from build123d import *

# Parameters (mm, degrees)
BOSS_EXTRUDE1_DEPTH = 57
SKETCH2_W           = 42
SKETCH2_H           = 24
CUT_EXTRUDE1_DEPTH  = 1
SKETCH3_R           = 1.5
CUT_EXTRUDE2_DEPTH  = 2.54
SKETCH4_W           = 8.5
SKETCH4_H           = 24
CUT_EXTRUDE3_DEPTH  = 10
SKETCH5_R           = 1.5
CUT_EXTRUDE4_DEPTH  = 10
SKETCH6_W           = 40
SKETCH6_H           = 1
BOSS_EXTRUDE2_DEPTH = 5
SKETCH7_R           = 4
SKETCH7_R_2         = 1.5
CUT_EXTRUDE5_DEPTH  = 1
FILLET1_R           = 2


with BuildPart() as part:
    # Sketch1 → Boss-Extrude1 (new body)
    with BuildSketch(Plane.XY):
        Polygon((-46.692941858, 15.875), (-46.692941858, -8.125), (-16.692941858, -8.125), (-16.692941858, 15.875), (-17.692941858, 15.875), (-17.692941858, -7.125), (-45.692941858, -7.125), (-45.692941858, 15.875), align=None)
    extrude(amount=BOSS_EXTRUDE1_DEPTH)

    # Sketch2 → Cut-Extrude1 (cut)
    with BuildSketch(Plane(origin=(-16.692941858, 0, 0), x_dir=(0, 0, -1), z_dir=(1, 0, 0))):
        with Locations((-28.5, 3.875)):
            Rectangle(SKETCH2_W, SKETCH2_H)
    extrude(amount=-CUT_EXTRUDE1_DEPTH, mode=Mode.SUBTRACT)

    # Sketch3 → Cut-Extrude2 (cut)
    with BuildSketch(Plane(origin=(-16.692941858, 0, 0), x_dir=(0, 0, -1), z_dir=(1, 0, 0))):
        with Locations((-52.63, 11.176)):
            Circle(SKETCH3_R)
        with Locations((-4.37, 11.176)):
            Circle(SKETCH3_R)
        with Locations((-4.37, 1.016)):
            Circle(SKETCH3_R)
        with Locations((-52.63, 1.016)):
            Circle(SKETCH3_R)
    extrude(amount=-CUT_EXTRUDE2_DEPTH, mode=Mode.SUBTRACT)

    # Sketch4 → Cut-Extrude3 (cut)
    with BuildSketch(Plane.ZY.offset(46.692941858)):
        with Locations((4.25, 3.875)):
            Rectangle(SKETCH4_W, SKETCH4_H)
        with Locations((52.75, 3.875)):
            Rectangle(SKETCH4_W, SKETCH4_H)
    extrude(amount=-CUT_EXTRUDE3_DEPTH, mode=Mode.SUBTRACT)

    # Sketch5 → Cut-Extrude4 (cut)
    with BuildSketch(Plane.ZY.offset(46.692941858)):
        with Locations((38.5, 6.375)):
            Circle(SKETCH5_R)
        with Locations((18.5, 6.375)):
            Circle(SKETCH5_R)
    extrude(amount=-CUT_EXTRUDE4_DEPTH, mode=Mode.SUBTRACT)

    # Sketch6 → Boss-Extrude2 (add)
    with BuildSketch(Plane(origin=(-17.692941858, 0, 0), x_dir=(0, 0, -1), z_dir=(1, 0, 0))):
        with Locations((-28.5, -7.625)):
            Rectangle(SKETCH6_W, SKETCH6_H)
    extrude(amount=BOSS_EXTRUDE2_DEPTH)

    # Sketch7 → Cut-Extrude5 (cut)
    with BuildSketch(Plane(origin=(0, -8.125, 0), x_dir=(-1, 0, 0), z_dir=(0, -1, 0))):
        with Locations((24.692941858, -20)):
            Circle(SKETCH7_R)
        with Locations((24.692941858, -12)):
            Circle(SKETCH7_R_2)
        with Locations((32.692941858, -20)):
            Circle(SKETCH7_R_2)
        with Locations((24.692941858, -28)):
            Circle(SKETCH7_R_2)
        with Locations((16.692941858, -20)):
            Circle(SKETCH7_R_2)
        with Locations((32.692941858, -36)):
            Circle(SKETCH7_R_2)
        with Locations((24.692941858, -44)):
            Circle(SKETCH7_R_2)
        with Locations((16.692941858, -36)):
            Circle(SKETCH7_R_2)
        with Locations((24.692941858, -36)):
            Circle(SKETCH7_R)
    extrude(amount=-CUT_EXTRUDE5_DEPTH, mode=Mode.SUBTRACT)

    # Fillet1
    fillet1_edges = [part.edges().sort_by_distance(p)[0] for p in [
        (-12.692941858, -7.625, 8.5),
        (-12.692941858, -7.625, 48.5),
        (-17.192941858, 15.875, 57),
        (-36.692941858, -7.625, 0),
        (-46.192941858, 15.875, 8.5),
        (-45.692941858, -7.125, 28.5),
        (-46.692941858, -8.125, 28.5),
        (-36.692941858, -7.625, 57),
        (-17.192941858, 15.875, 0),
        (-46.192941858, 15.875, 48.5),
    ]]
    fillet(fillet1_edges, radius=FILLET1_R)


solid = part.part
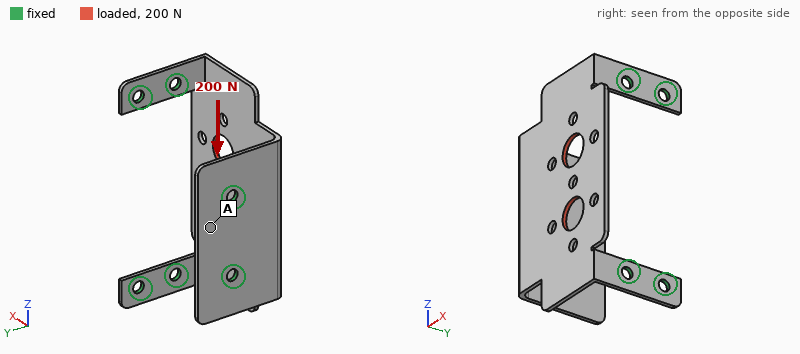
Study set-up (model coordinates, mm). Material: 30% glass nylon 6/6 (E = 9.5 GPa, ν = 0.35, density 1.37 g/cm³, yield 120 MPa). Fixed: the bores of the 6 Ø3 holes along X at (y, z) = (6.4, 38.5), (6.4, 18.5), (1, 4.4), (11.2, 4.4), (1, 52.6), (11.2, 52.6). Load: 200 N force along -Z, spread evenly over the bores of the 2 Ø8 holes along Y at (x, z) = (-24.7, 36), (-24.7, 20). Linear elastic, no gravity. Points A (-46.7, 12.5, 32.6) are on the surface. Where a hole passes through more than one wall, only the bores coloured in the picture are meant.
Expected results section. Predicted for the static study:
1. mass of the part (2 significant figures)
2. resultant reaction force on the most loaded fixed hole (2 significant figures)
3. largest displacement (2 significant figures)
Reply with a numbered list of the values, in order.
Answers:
1. 3.8 g
2. 89 N
3. 0.15 mm
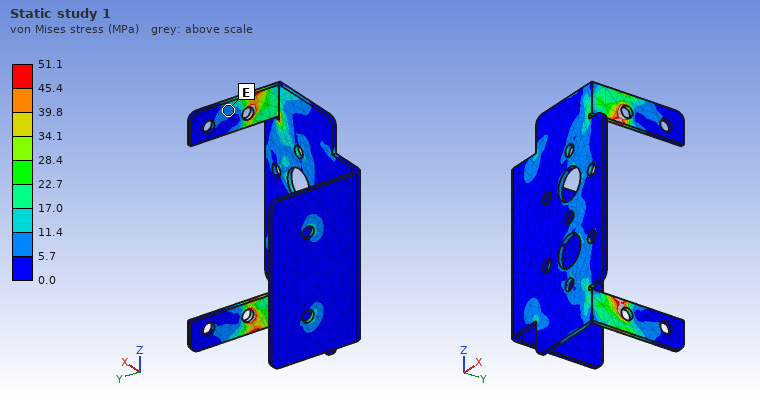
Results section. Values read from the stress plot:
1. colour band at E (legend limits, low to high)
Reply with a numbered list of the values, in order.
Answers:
1. 5.7 to 11.4 MPa
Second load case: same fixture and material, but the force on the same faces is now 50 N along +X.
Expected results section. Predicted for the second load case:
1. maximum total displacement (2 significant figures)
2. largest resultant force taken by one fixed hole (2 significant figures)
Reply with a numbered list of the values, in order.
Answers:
1. 0.24 mm
2. 17 N
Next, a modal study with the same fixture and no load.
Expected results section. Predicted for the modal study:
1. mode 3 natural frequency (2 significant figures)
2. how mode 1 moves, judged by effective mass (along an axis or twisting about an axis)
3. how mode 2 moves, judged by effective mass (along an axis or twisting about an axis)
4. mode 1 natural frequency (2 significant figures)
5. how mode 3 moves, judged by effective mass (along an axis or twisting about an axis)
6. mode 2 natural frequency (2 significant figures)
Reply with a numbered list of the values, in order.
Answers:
1. 2100 Hz
2. along Y
3. along X
4. 1200 Hz
5. along Y
6. 1600 Hz
